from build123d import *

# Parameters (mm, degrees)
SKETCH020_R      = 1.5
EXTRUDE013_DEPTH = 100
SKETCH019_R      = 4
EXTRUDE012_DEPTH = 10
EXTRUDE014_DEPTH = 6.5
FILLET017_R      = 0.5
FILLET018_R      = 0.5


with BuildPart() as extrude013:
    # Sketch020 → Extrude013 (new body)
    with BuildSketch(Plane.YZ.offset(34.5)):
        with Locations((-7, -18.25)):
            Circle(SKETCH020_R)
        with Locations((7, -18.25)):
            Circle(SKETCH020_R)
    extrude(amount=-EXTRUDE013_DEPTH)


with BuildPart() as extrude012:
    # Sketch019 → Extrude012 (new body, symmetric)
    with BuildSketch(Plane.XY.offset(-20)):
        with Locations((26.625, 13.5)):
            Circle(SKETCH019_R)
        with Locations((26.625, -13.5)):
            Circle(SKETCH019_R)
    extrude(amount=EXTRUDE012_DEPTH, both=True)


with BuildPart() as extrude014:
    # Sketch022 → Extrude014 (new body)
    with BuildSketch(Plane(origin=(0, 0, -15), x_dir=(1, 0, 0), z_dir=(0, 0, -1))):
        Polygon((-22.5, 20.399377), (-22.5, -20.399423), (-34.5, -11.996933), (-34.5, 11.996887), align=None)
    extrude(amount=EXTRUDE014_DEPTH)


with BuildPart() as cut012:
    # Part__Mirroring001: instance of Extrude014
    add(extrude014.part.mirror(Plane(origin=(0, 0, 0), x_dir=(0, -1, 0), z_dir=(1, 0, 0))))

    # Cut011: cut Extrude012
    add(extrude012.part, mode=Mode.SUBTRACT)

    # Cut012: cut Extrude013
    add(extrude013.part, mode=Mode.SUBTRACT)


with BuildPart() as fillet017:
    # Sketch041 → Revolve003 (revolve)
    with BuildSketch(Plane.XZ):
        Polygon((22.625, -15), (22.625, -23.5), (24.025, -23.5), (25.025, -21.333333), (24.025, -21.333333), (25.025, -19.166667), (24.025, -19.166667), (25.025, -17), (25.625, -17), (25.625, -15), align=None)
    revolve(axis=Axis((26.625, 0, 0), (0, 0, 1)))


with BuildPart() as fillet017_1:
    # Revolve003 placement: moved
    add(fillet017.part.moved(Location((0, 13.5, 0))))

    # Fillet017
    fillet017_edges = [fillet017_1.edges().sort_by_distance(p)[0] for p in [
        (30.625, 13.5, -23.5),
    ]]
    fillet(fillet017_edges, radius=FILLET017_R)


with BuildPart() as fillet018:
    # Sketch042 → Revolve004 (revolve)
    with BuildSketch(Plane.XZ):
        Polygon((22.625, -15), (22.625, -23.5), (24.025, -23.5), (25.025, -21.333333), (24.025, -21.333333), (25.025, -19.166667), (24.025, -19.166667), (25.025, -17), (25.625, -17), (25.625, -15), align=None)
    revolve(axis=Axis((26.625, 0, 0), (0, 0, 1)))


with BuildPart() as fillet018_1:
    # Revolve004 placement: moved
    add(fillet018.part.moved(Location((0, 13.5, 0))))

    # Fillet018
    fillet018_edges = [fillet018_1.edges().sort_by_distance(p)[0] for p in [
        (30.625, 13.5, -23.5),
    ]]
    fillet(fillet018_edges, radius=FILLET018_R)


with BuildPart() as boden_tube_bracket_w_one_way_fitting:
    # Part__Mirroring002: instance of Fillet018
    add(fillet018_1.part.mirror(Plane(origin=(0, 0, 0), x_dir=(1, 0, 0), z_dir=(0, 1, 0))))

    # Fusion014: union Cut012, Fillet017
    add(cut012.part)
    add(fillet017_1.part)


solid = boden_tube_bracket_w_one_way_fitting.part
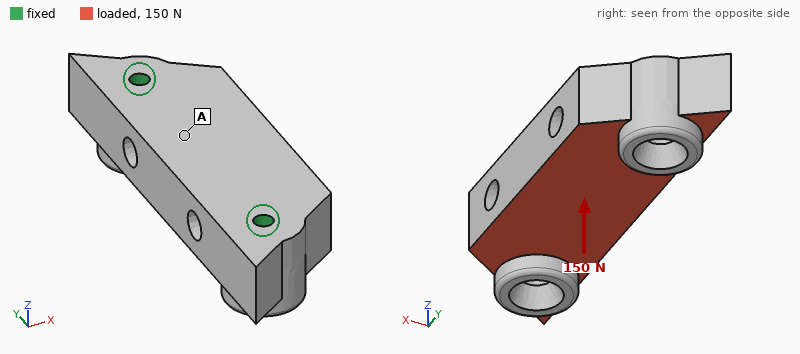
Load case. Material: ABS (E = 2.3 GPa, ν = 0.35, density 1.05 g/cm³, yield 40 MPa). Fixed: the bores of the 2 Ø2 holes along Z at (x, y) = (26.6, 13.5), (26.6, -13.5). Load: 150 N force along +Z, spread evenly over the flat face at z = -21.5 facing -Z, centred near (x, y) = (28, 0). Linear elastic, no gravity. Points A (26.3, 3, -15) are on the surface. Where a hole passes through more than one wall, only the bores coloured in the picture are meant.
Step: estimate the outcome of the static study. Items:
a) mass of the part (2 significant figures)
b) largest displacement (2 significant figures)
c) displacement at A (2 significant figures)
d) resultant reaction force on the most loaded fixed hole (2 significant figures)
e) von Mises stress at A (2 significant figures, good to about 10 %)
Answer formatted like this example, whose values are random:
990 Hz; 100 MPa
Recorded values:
2.5 g; 0.14 mm; 0.052 mm; 89 N; 2.9 MPa
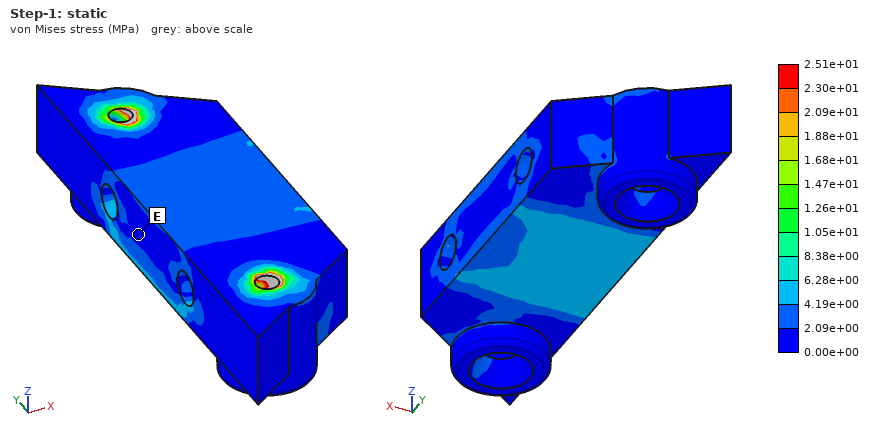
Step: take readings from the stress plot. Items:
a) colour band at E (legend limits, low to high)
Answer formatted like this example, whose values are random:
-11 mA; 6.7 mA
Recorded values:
0.00e+00 to 2.09e+00 MPa
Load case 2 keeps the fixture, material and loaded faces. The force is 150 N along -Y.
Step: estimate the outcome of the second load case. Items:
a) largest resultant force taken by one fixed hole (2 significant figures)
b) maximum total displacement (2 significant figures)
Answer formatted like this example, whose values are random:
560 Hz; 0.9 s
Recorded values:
81 N; 25 µm
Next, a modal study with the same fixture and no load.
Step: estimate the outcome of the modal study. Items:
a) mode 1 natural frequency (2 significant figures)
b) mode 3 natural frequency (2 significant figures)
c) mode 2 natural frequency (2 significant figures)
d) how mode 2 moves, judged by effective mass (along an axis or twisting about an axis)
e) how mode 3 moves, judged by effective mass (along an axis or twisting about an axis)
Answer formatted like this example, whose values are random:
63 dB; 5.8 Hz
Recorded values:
3600 Hz; 8700 Hz; 6600 Hz; along Z; along X
